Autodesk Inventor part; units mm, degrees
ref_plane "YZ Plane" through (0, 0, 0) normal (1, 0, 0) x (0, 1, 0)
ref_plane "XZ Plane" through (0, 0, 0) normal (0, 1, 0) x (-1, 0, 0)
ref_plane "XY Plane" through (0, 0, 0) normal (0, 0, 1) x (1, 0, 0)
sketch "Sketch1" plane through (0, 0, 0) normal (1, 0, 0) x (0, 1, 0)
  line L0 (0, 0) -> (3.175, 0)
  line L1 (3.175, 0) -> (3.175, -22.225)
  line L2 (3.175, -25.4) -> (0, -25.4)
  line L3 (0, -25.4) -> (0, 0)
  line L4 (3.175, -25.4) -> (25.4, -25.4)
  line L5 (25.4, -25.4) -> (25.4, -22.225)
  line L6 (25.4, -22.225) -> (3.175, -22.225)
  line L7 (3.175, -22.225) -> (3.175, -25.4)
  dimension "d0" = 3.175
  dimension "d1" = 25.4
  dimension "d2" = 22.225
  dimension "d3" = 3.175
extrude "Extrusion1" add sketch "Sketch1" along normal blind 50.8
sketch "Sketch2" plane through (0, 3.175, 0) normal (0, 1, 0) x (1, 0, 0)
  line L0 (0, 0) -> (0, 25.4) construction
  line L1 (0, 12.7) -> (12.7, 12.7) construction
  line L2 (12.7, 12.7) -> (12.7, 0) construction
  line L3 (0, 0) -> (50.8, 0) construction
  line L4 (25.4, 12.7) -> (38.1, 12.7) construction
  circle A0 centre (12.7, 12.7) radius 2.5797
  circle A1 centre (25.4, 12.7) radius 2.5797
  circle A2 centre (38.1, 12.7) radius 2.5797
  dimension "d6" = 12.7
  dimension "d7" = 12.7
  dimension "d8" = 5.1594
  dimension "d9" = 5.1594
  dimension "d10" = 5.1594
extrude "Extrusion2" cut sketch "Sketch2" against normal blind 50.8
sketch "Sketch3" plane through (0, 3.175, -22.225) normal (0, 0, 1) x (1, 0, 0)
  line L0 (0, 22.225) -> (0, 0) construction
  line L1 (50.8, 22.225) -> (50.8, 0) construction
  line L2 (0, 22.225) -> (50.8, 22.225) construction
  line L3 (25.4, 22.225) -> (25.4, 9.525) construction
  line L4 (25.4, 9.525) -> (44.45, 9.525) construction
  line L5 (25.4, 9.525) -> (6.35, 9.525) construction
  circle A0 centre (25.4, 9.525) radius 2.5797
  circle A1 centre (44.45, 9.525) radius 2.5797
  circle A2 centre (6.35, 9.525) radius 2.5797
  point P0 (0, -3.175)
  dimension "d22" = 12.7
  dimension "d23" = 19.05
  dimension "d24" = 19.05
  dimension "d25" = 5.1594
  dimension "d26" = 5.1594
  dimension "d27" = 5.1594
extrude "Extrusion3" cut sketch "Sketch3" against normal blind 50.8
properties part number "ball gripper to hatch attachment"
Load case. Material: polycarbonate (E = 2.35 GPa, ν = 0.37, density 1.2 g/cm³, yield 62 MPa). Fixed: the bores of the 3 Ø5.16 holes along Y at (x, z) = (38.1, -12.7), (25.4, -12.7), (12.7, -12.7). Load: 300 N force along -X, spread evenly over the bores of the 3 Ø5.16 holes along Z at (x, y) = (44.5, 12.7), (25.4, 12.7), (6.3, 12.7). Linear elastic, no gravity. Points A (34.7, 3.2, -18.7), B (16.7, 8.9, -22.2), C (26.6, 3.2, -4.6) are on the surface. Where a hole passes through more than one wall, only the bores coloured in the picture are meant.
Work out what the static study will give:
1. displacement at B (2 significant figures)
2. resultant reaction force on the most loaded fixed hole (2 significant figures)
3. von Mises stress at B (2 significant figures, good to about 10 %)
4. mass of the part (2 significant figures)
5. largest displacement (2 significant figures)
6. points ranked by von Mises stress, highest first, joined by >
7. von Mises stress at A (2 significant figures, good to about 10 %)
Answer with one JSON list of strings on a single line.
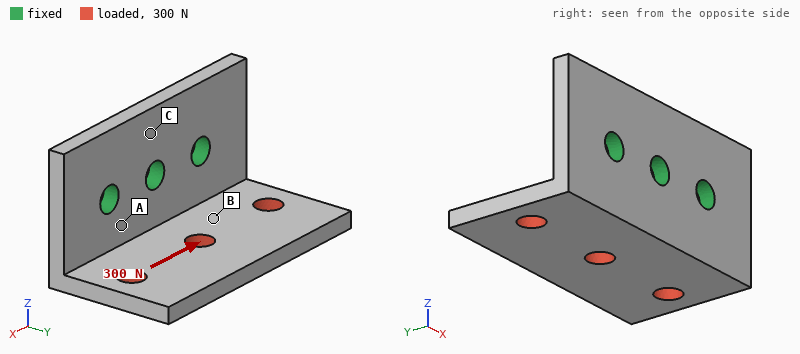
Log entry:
["0.20 mm", "180 N", "8.5 MPa", "8.7 g", "0.67 mm", "A > B > C", "13 MPa"]
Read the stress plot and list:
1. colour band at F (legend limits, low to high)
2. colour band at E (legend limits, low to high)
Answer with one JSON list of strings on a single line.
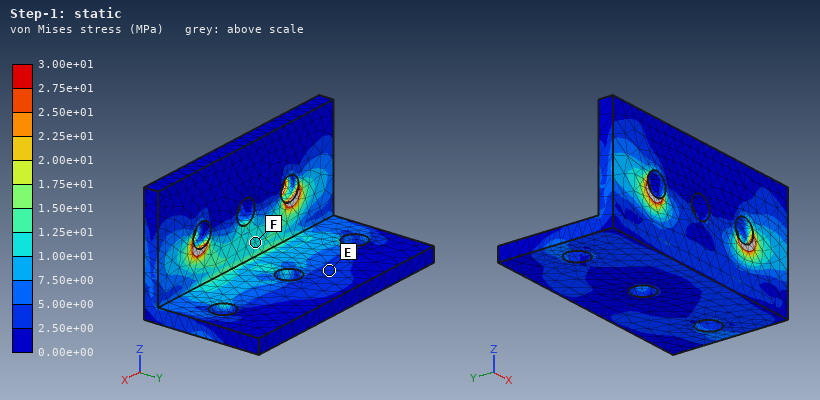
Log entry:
["1.00e+01 to 1.25e+01 MPa", "2.50e+00 to 5.00e+00 MPa"]
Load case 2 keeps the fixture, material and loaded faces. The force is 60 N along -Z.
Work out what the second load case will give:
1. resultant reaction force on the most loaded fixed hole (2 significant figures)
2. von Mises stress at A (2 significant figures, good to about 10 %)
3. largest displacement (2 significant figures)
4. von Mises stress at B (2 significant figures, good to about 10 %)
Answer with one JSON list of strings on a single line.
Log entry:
["24 N", "7.7 MPa", "0.65 mm", "2.7 MPa"]
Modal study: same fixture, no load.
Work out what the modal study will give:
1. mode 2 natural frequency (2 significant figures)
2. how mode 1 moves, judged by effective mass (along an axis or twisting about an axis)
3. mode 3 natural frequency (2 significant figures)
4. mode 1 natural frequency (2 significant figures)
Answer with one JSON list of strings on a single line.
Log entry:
["1300 Hz", "along Z", "2100 Hz", "800 Hz"]
